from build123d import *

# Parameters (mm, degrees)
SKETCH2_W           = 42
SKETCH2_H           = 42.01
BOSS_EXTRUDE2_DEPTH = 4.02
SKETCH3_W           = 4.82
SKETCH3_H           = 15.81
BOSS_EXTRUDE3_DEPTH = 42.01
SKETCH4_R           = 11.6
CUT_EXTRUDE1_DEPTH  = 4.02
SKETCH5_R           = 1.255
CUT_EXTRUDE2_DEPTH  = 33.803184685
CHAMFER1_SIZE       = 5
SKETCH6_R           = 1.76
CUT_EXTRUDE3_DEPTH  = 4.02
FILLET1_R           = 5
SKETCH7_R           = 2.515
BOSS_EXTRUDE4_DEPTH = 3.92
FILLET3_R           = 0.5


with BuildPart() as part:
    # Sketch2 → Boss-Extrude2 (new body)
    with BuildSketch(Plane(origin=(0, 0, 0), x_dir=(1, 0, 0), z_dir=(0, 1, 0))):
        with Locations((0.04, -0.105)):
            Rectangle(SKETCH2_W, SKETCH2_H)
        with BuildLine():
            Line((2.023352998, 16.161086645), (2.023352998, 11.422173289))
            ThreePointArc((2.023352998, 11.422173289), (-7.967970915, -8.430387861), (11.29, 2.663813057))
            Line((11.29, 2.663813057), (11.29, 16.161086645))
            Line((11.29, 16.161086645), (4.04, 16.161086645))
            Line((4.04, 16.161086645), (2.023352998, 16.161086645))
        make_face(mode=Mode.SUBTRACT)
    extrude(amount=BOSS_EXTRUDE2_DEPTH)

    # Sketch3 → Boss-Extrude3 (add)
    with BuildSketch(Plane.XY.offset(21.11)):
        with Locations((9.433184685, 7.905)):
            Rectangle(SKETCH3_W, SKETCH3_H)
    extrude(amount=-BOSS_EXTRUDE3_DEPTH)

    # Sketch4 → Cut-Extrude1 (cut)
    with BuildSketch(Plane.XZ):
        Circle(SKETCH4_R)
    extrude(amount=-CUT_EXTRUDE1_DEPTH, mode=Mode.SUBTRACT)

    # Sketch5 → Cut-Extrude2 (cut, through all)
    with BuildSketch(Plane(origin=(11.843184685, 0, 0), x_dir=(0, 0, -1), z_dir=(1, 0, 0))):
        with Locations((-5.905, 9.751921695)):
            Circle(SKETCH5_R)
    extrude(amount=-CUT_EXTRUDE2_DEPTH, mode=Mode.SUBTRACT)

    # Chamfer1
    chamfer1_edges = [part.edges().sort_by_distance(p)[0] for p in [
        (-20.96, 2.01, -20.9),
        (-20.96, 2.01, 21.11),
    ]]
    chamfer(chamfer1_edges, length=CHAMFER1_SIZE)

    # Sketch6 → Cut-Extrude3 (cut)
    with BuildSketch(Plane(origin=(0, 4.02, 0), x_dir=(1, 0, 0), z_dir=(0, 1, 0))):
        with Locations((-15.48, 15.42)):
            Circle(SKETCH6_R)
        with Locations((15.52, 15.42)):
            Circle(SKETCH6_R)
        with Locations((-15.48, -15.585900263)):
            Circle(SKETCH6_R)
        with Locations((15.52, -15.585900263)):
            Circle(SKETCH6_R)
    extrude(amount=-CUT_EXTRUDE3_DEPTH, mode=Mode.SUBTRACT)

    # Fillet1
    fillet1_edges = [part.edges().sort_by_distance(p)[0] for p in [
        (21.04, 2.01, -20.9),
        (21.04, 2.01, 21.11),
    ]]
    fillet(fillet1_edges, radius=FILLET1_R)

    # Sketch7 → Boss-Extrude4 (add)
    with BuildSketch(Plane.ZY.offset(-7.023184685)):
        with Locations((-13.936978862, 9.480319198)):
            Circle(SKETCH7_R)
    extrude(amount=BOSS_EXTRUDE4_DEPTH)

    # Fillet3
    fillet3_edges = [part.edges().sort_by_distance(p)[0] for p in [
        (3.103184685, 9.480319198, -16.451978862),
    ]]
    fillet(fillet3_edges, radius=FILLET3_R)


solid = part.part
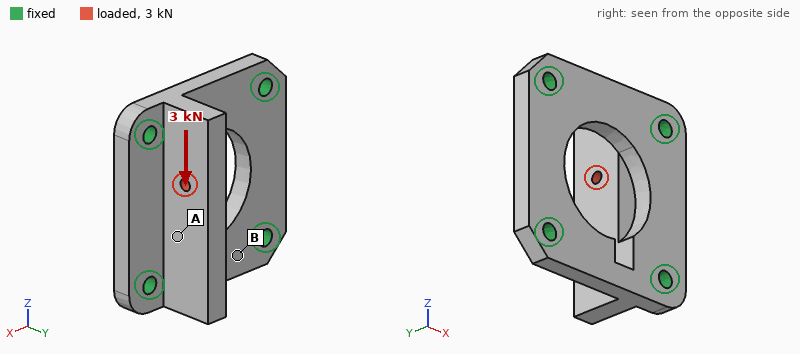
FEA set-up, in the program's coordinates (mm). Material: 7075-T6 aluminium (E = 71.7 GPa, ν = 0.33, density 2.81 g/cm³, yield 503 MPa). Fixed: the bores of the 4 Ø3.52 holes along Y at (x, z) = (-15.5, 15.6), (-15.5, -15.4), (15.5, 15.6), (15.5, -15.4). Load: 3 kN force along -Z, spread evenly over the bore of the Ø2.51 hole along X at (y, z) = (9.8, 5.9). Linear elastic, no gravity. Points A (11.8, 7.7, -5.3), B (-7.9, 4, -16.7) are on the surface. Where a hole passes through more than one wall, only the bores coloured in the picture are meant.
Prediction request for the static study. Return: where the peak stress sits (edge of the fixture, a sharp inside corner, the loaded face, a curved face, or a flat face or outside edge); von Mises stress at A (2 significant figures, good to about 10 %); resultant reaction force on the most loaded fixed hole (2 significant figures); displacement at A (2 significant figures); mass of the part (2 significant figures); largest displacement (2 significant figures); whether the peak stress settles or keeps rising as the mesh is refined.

edge of the fixture
37 MPa
1.7 kN
10 µm
21 g
21 µm
keeps rising
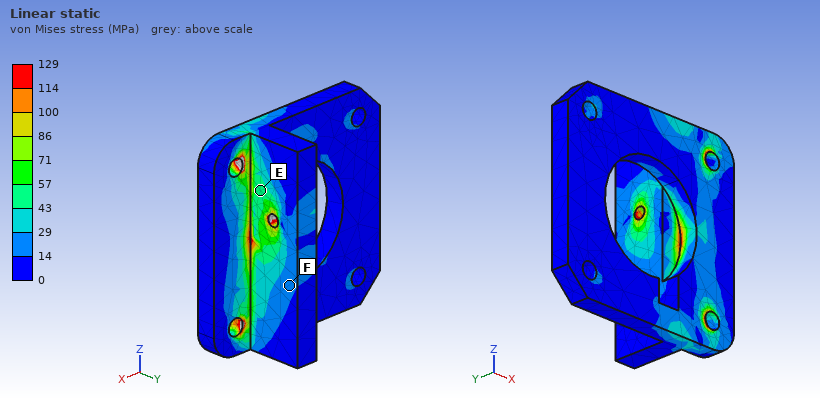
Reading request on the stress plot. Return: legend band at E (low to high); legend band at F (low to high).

43 to 57 MPa
14 to 29 MPa
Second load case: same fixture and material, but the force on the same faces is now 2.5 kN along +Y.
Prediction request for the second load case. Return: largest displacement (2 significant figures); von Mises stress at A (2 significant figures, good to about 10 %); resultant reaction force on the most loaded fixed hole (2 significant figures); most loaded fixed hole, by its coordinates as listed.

54 µm
23 MPa
1.6 kN
(15.5, 15.6)
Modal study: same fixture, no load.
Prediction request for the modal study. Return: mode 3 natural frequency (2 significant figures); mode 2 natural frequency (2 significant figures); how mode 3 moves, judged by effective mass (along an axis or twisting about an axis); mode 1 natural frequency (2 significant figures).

22 kHz
16 kHz
along Y
10000 Hz
